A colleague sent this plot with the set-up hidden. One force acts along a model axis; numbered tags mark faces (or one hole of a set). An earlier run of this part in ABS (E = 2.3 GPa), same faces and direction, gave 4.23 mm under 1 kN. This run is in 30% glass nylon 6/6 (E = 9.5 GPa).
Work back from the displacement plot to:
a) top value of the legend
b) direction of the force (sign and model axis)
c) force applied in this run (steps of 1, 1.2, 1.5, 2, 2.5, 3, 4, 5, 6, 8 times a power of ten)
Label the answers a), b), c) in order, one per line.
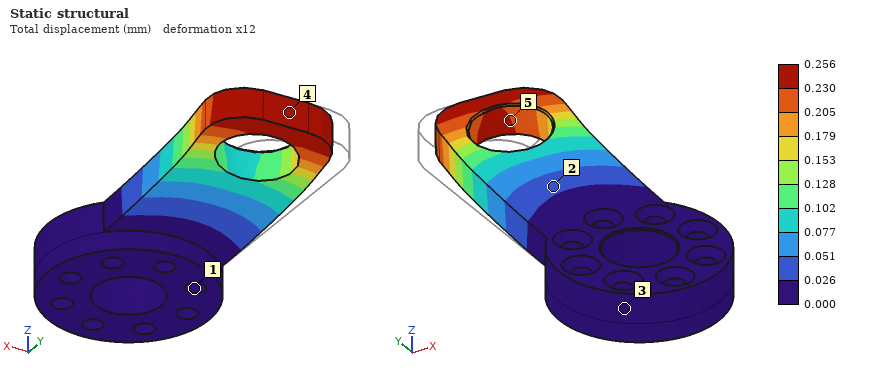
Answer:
a) 0.256 mm
b) +X
c) 250 N
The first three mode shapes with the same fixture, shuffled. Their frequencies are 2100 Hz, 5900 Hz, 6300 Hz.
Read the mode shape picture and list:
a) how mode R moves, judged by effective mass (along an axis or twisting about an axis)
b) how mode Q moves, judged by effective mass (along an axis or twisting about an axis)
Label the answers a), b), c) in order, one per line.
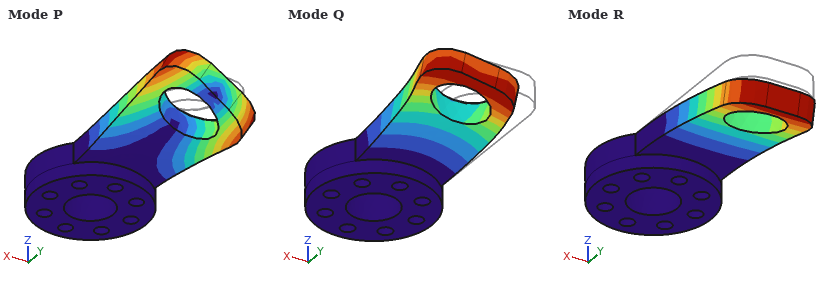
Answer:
a) along Z
b) along X
